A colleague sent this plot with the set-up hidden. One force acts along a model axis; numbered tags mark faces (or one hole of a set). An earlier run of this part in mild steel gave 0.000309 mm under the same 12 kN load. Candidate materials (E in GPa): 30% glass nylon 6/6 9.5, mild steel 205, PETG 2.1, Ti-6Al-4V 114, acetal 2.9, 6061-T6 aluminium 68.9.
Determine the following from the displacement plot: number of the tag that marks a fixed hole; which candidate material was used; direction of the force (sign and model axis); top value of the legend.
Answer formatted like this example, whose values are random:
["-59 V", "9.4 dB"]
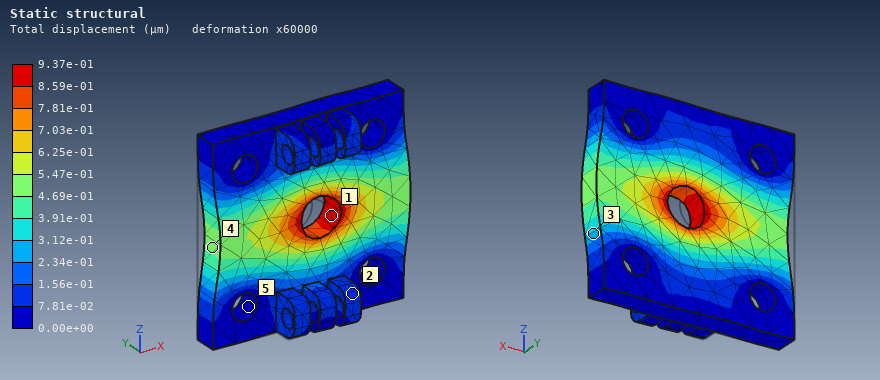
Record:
["5", "6061-T6 aluminium", "+X", "9.37e-01 µm"]
